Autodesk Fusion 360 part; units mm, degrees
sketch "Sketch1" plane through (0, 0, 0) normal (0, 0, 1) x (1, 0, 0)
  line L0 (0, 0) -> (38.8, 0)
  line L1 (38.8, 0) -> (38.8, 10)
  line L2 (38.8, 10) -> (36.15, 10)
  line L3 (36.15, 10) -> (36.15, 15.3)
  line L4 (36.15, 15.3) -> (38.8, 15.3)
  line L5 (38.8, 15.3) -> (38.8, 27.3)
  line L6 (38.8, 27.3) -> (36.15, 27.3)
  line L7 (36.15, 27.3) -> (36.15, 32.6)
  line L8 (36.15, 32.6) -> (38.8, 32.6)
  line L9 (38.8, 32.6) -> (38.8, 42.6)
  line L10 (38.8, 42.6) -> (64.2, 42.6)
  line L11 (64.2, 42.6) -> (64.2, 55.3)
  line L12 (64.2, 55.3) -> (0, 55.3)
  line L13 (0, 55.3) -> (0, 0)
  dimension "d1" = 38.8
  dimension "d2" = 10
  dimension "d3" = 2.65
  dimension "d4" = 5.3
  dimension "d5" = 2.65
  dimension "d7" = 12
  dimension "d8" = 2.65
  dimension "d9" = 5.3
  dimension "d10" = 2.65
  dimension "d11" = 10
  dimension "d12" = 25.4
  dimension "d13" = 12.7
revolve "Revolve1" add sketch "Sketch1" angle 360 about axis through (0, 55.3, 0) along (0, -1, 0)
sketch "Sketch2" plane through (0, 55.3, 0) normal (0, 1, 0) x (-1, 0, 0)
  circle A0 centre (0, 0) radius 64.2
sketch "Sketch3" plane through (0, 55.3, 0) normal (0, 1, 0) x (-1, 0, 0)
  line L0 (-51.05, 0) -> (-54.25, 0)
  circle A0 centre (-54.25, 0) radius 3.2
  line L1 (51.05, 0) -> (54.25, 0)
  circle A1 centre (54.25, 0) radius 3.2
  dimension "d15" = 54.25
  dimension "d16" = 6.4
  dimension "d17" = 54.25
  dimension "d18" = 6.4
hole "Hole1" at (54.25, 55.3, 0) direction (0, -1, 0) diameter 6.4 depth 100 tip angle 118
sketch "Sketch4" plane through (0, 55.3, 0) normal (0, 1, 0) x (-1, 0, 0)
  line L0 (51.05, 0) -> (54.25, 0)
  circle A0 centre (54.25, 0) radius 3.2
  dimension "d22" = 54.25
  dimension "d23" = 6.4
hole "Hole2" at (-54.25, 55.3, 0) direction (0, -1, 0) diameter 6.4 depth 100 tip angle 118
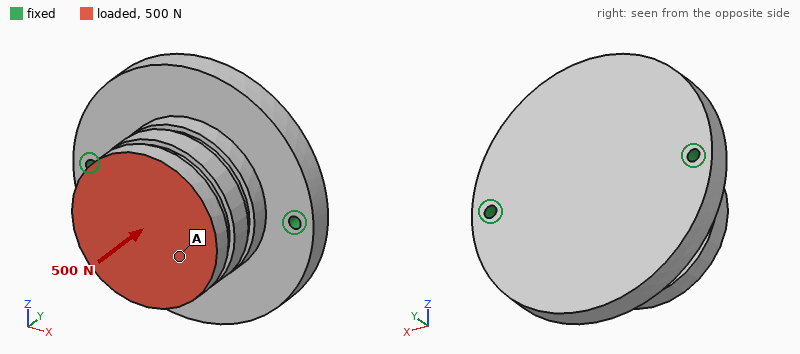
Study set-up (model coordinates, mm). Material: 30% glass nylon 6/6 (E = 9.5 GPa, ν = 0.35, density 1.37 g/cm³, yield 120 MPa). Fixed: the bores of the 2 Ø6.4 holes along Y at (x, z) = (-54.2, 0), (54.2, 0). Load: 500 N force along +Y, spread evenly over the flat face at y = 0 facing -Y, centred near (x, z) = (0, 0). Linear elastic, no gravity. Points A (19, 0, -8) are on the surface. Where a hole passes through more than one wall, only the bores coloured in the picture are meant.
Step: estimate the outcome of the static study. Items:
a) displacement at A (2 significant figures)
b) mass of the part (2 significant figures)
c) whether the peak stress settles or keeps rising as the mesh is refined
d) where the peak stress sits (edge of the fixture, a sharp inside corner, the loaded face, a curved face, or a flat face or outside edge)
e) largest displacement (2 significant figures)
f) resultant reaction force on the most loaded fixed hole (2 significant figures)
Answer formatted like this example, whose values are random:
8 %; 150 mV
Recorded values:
9.8 µm; 490 g; keeps rising; edge of the fixture; 12 µm; 270 N
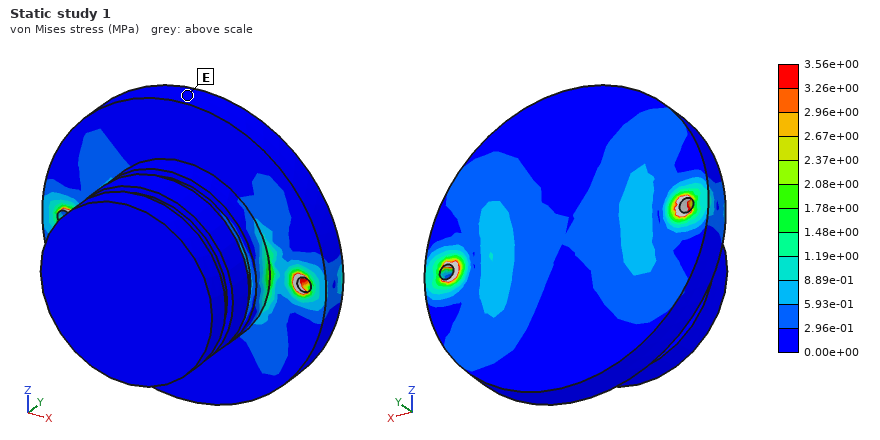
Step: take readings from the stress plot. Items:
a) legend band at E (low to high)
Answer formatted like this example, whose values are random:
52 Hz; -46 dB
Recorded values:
0.00e+00 to 2.96e-01 MPa
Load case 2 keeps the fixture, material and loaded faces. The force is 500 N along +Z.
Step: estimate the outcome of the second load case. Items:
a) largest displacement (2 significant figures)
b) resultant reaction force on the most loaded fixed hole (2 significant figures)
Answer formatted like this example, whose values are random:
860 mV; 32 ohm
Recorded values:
0.17 mm; 250 N
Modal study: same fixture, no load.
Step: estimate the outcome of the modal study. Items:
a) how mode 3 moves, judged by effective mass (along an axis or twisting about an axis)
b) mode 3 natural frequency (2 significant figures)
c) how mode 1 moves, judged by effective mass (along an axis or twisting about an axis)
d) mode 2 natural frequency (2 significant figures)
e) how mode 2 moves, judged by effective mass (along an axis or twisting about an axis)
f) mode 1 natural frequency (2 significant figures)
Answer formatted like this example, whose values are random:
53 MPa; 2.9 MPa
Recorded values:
along X; 2500 Hz; along Z; 1700 Hz; along Y; 640 Hz
